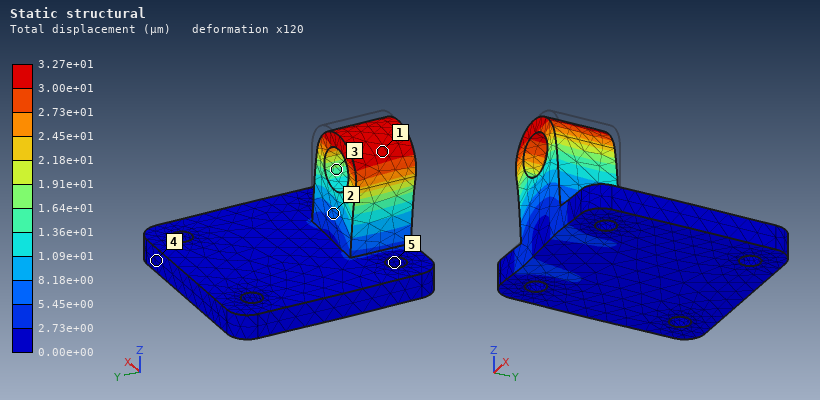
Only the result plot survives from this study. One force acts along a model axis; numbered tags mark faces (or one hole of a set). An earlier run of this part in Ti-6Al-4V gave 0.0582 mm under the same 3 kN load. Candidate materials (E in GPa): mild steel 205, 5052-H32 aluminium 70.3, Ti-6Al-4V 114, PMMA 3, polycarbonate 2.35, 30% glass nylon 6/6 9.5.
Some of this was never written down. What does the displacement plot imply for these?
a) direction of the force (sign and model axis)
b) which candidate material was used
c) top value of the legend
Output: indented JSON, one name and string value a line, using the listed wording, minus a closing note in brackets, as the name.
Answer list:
{
  "direction of the force": "-X",
  "which candidate material was used": "mild steel",
  "top value of the legend": "3.27e+01 µm"
}
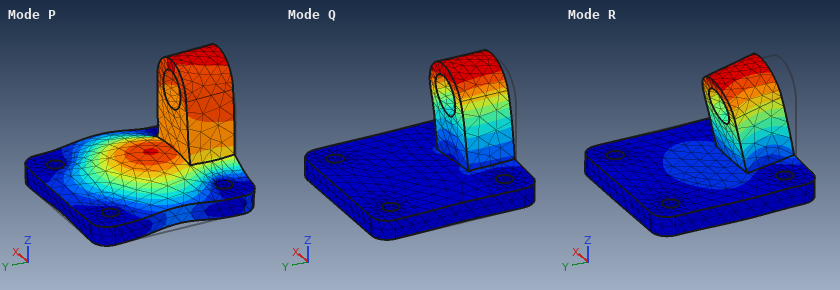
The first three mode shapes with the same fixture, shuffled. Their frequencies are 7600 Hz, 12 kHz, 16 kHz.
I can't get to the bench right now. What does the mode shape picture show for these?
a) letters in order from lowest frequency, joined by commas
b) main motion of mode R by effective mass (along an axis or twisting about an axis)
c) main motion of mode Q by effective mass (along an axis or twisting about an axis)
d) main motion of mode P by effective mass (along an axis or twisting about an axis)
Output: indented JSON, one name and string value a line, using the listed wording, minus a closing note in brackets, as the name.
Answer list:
{
  "letters in order from lowest frequency, joined by commas": "R, Q, P",
  "main motion of mode R by effective mass": "along Y",
  "main motion of mode Q by effective mass": "along X",
  "main motion of mode P by effective mass": "along Z"
}
